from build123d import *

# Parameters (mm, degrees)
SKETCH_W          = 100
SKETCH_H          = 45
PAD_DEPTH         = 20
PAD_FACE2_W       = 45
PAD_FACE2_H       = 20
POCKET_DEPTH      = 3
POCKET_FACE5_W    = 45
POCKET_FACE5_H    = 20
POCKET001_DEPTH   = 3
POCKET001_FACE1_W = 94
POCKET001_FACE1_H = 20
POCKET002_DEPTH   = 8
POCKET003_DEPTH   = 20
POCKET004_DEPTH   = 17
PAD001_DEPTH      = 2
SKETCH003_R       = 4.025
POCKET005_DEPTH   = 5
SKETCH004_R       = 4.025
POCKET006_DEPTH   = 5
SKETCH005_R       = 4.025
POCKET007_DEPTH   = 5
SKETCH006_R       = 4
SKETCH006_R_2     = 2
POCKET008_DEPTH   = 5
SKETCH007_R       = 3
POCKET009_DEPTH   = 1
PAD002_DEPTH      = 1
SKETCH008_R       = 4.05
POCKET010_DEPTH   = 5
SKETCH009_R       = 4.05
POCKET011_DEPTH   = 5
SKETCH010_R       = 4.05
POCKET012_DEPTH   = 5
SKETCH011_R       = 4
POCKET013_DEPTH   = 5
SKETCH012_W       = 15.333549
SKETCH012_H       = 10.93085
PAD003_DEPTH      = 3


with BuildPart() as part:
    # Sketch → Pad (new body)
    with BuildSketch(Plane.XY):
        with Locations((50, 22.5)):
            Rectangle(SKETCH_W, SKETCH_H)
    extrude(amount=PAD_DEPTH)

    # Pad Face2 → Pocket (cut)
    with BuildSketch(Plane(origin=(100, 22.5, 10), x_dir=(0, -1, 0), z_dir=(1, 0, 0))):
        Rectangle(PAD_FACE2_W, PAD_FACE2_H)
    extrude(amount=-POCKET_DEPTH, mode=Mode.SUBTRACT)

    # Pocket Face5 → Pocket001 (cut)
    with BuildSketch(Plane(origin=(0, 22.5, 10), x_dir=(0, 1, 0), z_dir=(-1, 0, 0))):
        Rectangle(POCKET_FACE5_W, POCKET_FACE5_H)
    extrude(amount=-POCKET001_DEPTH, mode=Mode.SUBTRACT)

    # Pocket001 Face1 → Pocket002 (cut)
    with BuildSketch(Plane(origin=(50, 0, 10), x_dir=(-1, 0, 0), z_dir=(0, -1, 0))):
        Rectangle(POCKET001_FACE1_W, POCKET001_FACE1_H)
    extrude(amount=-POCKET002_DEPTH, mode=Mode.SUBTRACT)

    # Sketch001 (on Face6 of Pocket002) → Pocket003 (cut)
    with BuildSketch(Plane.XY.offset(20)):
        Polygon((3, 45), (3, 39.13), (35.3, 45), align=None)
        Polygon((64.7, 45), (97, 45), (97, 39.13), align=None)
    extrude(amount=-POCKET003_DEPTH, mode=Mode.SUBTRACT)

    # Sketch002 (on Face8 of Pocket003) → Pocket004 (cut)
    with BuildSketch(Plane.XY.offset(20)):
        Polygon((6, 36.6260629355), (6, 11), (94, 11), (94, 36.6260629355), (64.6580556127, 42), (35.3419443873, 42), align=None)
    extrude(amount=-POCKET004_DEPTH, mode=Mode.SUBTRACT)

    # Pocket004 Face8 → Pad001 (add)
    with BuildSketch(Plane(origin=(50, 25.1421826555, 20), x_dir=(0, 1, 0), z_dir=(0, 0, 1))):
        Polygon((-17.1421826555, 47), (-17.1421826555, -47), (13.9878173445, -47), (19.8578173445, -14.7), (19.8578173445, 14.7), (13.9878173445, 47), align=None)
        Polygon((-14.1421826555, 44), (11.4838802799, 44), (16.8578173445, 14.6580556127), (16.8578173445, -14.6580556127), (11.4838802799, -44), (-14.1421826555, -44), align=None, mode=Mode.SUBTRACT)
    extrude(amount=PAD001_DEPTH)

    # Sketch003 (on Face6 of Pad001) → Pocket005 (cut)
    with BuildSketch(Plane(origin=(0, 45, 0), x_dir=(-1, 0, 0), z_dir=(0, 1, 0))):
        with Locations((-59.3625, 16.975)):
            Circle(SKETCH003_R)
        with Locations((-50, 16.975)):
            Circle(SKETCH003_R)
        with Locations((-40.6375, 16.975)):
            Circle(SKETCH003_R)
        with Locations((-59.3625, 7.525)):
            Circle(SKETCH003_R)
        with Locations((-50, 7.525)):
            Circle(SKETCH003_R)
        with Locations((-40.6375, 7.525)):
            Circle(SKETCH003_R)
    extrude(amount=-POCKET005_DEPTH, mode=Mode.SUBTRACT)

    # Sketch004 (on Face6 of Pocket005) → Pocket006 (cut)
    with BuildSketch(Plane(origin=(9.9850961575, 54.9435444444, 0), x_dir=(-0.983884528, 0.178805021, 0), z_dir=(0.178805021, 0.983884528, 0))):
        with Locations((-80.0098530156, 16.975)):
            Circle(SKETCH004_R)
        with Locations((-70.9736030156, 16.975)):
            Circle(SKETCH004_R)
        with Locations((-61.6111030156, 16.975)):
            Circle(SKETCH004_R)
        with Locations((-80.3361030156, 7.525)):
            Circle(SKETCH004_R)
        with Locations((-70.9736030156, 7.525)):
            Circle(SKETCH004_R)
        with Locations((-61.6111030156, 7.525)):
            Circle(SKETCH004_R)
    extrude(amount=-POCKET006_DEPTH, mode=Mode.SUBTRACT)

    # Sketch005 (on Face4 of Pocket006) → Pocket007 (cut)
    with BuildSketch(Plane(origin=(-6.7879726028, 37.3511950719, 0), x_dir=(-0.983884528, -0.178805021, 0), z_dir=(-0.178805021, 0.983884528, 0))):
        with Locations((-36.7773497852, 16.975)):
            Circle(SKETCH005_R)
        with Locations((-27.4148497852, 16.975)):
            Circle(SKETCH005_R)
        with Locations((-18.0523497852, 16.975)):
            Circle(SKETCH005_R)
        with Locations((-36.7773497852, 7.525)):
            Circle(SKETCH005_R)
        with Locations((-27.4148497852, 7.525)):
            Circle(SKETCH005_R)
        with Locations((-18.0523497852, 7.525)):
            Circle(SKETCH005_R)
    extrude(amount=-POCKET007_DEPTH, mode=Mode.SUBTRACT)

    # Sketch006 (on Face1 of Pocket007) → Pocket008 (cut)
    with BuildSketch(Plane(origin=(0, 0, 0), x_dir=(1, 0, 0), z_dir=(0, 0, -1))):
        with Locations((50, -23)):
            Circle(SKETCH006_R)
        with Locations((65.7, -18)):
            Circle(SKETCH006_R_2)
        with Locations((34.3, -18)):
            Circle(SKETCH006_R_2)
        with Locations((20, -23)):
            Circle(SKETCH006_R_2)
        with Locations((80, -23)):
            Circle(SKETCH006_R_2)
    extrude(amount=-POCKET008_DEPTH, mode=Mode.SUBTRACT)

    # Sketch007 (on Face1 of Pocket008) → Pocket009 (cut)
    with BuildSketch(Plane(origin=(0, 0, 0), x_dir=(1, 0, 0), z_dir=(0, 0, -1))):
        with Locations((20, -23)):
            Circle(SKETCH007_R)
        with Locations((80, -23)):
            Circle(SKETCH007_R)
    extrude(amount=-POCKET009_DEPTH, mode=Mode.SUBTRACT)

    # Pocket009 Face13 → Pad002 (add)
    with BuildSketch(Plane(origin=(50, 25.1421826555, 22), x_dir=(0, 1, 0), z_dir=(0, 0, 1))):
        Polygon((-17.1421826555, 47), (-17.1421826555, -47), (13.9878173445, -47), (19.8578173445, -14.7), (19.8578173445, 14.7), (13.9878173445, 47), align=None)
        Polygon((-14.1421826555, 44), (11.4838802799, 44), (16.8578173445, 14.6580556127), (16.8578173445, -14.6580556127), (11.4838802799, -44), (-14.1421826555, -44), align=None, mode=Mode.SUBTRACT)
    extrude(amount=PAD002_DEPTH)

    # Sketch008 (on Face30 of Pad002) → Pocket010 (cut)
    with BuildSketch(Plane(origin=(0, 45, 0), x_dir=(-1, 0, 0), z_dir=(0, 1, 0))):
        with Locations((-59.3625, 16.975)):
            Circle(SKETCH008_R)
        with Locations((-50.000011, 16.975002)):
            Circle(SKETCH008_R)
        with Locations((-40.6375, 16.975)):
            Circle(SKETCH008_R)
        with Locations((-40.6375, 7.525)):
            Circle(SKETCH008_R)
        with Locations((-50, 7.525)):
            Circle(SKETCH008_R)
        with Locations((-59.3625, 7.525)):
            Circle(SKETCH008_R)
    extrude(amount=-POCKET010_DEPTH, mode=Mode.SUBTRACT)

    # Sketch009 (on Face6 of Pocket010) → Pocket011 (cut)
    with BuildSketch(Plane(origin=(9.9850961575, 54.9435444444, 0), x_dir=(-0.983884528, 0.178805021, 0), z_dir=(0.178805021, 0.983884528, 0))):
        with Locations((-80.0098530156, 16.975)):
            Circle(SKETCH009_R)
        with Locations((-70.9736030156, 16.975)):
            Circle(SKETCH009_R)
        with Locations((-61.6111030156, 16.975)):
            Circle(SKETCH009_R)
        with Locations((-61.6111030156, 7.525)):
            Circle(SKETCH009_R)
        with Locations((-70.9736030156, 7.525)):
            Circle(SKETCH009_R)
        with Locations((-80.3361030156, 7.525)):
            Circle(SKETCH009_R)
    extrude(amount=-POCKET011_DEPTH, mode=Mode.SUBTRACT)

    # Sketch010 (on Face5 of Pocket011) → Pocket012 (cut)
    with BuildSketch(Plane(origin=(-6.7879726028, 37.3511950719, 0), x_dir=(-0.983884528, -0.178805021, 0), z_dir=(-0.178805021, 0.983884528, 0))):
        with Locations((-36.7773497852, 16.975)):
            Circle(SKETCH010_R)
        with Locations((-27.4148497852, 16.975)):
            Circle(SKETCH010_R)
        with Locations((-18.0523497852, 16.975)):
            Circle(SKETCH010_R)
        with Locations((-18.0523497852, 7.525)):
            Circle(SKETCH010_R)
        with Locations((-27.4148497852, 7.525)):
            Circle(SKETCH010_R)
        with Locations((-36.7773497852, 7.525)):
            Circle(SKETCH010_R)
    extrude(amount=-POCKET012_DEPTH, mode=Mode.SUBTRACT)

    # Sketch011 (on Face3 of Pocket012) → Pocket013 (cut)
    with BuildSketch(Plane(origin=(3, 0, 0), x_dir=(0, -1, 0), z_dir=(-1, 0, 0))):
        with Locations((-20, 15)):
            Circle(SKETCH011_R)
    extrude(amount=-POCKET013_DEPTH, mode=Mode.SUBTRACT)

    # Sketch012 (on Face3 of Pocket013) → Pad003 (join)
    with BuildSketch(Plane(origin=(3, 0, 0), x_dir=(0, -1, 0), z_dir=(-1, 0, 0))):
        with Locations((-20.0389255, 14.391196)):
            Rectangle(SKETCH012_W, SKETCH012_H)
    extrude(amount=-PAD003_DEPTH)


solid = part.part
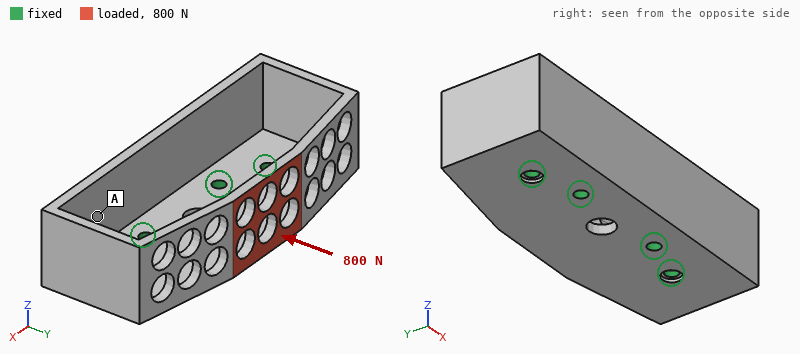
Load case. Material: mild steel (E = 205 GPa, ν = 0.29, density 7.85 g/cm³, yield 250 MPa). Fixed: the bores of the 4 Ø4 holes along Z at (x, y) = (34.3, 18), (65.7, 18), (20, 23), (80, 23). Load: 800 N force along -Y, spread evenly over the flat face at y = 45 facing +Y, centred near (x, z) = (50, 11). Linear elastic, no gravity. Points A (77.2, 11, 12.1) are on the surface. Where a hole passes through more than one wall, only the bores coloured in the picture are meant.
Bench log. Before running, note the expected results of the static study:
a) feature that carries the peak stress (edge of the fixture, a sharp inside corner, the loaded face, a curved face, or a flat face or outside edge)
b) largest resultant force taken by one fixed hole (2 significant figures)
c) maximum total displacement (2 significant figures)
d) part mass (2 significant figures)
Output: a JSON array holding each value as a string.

["a curved face", "300 N", "0.17 mm", "170 g"]
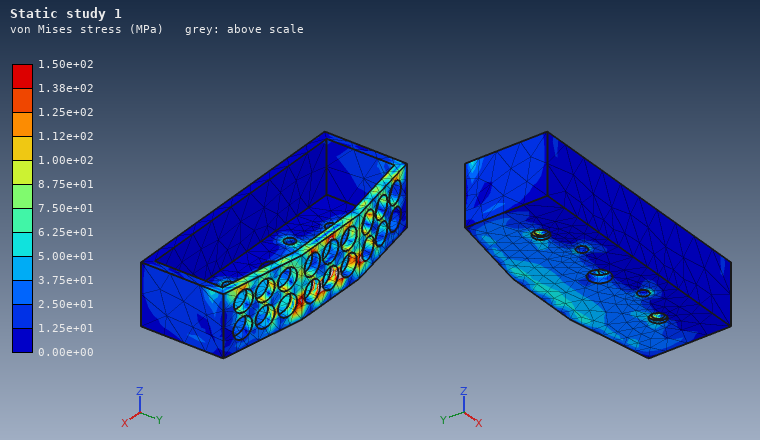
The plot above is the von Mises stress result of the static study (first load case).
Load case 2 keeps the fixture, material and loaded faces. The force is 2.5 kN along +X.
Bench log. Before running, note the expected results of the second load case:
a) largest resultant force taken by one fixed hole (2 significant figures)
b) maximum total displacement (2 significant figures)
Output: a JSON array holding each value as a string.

["1.3 kN", "56 µm"]
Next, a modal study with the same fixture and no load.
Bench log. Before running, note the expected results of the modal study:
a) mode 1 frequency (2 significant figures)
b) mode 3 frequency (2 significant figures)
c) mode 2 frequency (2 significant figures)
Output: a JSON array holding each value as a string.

["2500 Hz", "3800 Hz", "2800 Hz"]
